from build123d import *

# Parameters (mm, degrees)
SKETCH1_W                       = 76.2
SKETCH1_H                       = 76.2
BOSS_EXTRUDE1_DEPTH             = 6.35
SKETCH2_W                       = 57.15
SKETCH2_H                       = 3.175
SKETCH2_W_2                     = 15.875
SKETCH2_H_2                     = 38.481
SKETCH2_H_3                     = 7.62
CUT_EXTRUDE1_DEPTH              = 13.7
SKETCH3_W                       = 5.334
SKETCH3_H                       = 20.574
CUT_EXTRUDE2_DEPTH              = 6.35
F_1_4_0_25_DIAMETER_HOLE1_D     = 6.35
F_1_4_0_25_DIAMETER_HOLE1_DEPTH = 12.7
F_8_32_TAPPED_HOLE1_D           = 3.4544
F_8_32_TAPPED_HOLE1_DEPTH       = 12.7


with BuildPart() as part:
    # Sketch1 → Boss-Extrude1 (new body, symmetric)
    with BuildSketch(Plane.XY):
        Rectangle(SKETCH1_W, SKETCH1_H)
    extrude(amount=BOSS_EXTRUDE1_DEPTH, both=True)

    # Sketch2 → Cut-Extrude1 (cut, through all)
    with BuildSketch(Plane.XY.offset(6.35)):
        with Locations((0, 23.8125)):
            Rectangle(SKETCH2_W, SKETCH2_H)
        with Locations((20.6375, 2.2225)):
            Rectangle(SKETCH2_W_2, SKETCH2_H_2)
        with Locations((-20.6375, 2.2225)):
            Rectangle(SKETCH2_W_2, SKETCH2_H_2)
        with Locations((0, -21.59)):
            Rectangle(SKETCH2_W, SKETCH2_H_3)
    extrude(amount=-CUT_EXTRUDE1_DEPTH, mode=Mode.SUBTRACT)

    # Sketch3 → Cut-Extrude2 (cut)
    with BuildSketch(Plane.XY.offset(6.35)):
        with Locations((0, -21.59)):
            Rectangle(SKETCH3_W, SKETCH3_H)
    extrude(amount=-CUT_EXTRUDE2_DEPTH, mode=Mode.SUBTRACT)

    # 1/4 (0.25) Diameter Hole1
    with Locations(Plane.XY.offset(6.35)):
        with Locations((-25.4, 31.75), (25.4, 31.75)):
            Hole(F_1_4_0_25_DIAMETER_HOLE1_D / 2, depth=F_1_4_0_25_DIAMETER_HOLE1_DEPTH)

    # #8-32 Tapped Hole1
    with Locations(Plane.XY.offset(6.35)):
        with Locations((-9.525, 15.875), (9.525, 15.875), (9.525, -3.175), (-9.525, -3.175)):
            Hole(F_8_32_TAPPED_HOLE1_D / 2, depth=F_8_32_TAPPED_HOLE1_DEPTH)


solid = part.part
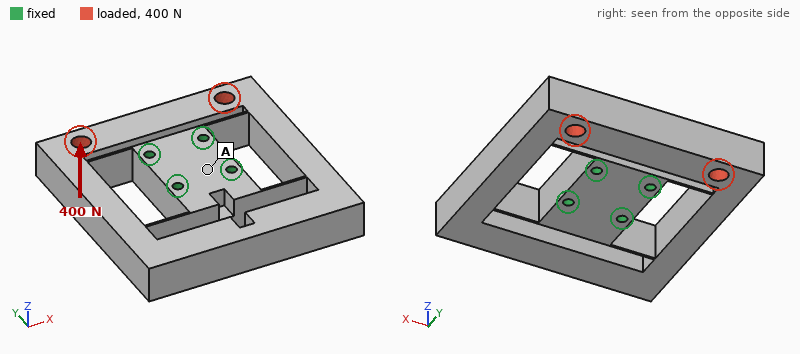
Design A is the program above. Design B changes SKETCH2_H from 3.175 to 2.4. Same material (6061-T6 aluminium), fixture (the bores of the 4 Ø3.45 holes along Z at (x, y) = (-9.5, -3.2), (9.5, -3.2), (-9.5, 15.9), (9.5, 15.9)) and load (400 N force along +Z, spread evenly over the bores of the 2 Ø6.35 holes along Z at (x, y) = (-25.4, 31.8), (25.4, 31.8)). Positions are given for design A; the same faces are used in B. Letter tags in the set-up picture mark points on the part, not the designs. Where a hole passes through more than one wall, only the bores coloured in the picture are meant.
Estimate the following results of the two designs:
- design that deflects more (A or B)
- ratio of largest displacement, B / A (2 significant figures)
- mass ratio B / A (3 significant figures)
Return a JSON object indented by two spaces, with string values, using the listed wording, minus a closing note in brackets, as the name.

{
  "design that deflects more": "A",
  "ratio of largest displacement, B / A": "0.78",
  "mass ratio B / A": "1.01"
}
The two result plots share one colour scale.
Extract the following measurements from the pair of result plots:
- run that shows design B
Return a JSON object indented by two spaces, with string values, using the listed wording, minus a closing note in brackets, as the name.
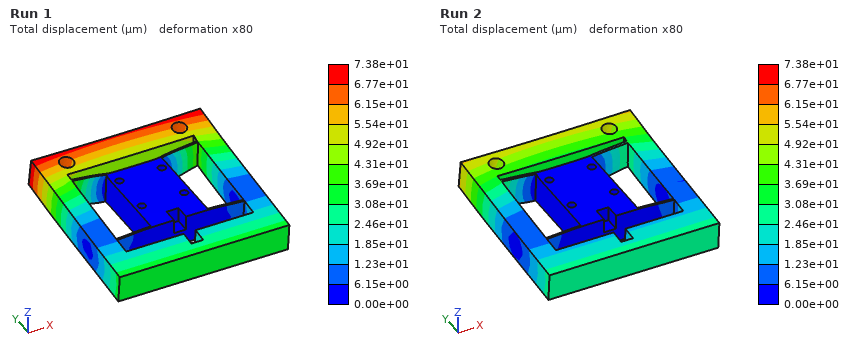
{
  "run that shows design B": "Run 2"
}
